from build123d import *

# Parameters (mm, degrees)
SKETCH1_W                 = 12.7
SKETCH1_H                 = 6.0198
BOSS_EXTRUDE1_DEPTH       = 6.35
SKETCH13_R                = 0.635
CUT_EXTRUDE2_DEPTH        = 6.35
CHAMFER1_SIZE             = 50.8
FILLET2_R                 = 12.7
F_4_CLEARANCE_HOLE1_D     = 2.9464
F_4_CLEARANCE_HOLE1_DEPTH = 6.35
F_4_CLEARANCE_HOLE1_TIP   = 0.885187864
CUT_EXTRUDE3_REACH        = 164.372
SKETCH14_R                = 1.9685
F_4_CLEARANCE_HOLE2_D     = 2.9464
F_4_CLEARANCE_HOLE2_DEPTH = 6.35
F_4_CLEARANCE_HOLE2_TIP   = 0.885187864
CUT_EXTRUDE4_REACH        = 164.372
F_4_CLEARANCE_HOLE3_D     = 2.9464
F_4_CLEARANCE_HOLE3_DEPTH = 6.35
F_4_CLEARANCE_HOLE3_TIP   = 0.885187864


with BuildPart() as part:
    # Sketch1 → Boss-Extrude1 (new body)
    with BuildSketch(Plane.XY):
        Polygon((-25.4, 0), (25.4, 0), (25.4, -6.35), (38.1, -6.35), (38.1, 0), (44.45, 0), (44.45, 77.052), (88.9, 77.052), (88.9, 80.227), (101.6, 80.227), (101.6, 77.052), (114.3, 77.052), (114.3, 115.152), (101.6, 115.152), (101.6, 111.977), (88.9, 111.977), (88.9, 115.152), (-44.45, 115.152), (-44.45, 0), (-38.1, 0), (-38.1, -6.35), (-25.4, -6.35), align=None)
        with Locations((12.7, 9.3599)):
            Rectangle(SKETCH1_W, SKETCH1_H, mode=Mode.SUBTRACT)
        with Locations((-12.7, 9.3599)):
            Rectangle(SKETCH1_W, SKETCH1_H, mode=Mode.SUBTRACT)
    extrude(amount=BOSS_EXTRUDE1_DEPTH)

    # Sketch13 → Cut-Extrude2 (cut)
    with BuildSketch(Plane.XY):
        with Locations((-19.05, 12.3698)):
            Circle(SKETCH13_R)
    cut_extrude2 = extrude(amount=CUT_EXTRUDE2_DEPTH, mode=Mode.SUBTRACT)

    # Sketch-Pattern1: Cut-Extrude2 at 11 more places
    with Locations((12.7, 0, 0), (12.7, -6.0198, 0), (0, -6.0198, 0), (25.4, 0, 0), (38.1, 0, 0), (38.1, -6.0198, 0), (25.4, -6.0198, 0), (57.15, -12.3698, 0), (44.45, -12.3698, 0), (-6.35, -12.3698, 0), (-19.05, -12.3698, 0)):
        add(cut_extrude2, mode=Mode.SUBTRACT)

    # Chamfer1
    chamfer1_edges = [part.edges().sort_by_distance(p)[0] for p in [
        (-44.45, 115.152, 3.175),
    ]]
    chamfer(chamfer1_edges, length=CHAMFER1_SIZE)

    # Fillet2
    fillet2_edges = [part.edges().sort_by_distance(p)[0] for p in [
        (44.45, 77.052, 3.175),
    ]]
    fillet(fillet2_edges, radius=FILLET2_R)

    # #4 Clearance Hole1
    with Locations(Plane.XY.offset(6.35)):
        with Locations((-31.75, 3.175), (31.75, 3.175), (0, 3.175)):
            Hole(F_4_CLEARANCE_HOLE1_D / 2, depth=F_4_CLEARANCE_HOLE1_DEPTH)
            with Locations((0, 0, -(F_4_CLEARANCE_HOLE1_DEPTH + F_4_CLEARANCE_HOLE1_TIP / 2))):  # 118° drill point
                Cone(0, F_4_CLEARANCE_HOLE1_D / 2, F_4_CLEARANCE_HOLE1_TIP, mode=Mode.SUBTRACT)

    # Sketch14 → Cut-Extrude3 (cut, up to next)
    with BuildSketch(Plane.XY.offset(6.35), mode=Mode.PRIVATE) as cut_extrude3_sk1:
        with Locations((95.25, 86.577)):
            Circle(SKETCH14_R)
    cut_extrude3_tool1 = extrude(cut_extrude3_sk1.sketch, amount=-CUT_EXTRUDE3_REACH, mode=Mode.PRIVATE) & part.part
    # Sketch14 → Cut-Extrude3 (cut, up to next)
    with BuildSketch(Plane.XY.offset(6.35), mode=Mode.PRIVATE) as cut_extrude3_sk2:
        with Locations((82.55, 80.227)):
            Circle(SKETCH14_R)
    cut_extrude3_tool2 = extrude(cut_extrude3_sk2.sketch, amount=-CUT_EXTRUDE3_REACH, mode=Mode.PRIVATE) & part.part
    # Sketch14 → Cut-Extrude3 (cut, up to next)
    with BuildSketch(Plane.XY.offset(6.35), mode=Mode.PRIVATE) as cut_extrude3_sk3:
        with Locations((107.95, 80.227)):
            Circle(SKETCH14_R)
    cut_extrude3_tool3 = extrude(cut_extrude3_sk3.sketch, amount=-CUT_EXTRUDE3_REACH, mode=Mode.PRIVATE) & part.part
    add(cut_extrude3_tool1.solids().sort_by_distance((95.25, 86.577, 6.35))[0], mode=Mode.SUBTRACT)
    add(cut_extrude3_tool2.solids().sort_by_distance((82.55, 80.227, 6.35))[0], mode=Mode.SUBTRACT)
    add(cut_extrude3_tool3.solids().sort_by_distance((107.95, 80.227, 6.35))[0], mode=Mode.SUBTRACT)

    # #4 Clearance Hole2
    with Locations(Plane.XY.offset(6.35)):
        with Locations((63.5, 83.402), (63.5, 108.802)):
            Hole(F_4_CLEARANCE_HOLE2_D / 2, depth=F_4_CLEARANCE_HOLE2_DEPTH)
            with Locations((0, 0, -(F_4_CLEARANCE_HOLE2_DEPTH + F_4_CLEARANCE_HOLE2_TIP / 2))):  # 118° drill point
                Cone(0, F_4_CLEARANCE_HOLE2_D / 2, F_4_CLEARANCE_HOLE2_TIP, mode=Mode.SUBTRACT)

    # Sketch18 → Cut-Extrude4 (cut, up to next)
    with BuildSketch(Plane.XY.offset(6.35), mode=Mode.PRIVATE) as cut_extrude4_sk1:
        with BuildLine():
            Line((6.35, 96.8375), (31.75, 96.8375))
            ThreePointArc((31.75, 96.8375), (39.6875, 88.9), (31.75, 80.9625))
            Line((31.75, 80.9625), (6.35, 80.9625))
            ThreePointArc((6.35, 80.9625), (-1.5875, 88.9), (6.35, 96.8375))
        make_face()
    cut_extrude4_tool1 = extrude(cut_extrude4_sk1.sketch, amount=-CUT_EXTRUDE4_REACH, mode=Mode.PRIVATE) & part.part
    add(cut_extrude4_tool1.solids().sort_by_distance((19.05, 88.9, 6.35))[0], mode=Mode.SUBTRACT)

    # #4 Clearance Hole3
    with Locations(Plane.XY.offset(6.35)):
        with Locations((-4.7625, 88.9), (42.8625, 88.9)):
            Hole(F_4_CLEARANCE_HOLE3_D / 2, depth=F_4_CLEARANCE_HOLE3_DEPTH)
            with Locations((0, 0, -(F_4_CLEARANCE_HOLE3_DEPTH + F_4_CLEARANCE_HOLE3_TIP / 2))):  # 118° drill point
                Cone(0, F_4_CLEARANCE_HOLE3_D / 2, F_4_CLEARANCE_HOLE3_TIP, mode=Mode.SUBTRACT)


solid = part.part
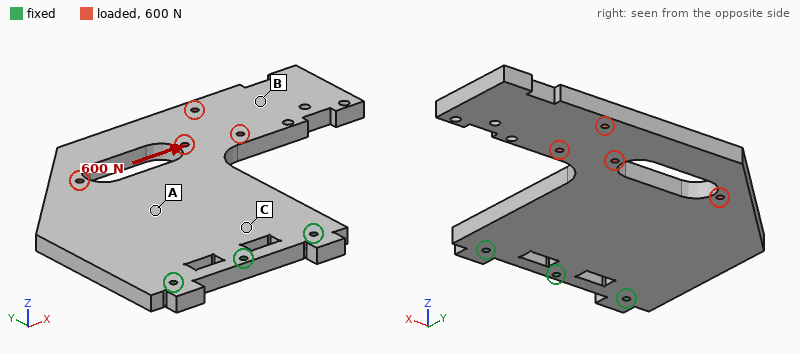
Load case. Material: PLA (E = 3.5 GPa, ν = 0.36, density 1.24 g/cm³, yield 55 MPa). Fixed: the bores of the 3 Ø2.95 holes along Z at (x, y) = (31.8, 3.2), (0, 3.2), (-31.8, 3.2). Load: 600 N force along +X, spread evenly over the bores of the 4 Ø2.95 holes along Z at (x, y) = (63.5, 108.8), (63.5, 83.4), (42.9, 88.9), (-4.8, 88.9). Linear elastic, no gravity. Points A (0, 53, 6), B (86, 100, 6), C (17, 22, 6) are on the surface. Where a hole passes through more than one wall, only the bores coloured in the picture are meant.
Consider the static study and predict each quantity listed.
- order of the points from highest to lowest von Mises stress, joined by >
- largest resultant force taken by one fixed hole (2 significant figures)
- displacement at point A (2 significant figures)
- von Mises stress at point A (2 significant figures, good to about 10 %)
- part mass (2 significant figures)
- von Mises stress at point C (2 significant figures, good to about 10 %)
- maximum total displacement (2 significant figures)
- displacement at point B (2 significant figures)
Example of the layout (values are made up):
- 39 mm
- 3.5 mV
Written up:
- C > A > B
- 850 N
- 0.14 mm
- 3.0 MPa
- 86 g
- 4.6 MPa
- 0.65 mm
- 0.51 mm
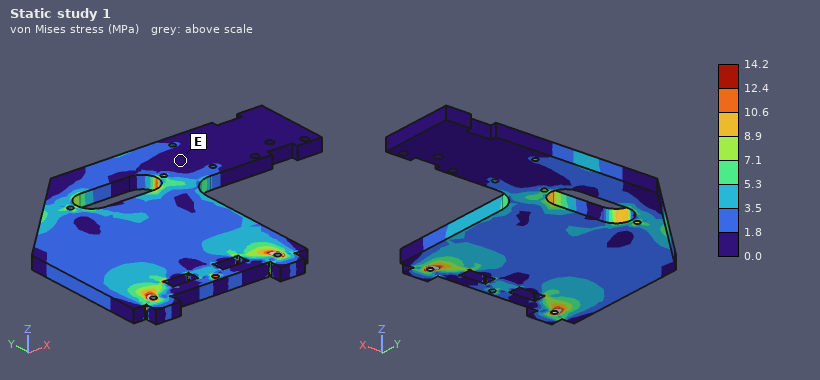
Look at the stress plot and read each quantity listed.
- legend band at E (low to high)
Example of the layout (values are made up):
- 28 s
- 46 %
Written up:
- 0.0 to 1.8 MPa
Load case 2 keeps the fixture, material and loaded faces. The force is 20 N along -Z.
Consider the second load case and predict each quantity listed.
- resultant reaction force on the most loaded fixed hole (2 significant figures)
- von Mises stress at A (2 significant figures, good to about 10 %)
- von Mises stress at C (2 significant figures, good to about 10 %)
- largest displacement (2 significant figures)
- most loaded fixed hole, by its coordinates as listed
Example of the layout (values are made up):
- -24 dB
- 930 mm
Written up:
- 18 N
- 1.6 MPa
- 1.9 MPa
- 2.3 mm
- (31.8, 3.2)
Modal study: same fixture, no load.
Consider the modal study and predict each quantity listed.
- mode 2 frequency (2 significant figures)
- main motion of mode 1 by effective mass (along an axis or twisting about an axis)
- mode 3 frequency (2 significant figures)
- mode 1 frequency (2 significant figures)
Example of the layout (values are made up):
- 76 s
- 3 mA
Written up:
- 210 Hz
- along Z
- 570 Hz
- 89 Hz
